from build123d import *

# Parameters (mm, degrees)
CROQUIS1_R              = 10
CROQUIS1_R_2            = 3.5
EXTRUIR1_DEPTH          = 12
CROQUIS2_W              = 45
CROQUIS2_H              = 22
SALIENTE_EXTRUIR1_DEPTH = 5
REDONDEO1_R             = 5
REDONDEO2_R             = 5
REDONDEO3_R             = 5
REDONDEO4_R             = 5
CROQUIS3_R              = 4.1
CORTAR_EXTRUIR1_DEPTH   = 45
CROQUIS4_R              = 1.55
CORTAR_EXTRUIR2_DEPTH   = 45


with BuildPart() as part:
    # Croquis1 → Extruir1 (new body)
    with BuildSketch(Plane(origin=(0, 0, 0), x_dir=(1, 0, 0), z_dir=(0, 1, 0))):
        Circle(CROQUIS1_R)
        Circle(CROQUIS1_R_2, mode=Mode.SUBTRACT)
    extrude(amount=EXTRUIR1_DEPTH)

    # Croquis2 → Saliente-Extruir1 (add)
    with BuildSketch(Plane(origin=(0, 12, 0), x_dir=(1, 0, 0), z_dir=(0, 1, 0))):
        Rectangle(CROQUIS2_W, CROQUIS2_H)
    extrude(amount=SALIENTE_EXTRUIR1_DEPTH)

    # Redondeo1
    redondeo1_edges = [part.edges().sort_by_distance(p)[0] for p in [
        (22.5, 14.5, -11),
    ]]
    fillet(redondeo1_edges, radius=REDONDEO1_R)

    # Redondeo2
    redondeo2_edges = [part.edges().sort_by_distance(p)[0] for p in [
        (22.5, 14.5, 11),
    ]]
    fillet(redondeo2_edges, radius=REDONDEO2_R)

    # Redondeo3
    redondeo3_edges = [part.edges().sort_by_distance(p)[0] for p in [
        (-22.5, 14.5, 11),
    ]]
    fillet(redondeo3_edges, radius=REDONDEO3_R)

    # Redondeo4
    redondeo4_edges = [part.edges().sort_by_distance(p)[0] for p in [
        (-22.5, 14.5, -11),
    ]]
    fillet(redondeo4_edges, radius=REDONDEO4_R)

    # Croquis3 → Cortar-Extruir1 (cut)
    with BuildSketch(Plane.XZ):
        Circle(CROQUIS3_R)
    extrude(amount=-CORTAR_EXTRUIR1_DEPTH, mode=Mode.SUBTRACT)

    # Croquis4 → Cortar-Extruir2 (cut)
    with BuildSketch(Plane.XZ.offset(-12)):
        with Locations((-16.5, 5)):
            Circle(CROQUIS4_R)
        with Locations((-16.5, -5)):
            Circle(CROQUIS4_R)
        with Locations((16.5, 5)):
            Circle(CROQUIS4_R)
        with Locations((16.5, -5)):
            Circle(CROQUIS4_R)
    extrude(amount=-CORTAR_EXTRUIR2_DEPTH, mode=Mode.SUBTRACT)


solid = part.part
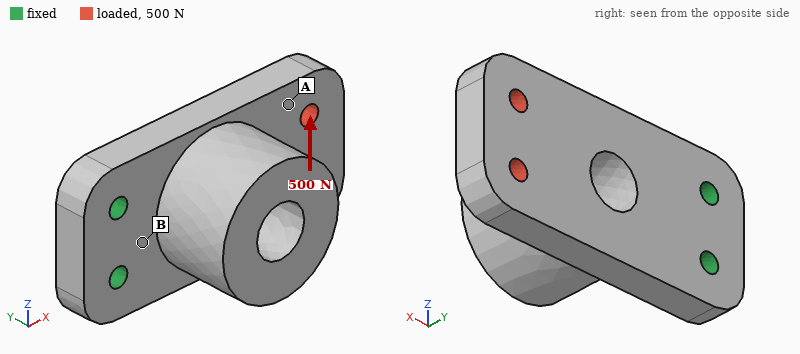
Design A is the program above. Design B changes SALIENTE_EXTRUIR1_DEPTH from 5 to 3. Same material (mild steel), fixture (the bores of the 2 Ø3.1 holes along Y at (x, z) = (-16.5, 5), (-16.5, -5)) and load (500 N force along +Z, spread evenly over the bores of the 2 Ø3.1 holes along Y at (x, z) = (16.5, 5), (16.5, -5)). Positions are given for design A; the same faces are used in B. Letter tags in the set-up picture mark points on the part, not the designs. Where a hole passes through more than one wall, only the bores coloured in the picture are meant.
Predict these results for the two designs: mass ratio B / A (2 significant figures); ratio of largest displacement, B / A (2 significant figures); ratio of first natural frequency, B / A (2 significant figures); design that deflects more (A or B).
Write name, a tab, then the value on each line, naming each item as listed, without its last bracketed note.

mass ratio B / A	0.77
ratio of largest displacement, B / A	1.6
ratio of first natural frequency, B / A	0.60
design that deflects more	B
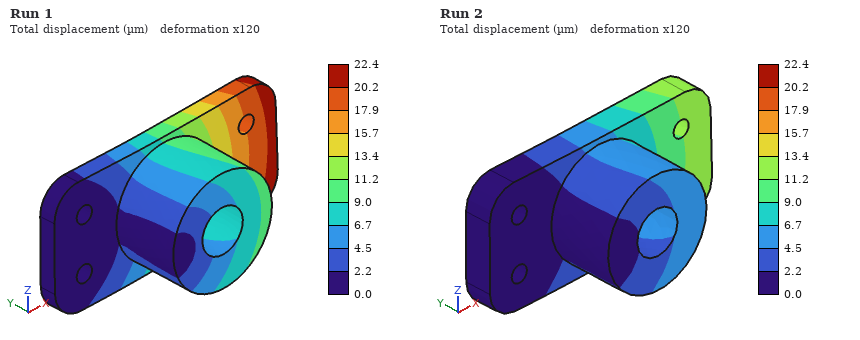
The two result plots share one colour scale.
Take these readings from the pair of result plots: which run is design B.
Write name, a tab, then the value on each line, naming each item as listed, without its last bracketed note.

which run is design B	Run 1
